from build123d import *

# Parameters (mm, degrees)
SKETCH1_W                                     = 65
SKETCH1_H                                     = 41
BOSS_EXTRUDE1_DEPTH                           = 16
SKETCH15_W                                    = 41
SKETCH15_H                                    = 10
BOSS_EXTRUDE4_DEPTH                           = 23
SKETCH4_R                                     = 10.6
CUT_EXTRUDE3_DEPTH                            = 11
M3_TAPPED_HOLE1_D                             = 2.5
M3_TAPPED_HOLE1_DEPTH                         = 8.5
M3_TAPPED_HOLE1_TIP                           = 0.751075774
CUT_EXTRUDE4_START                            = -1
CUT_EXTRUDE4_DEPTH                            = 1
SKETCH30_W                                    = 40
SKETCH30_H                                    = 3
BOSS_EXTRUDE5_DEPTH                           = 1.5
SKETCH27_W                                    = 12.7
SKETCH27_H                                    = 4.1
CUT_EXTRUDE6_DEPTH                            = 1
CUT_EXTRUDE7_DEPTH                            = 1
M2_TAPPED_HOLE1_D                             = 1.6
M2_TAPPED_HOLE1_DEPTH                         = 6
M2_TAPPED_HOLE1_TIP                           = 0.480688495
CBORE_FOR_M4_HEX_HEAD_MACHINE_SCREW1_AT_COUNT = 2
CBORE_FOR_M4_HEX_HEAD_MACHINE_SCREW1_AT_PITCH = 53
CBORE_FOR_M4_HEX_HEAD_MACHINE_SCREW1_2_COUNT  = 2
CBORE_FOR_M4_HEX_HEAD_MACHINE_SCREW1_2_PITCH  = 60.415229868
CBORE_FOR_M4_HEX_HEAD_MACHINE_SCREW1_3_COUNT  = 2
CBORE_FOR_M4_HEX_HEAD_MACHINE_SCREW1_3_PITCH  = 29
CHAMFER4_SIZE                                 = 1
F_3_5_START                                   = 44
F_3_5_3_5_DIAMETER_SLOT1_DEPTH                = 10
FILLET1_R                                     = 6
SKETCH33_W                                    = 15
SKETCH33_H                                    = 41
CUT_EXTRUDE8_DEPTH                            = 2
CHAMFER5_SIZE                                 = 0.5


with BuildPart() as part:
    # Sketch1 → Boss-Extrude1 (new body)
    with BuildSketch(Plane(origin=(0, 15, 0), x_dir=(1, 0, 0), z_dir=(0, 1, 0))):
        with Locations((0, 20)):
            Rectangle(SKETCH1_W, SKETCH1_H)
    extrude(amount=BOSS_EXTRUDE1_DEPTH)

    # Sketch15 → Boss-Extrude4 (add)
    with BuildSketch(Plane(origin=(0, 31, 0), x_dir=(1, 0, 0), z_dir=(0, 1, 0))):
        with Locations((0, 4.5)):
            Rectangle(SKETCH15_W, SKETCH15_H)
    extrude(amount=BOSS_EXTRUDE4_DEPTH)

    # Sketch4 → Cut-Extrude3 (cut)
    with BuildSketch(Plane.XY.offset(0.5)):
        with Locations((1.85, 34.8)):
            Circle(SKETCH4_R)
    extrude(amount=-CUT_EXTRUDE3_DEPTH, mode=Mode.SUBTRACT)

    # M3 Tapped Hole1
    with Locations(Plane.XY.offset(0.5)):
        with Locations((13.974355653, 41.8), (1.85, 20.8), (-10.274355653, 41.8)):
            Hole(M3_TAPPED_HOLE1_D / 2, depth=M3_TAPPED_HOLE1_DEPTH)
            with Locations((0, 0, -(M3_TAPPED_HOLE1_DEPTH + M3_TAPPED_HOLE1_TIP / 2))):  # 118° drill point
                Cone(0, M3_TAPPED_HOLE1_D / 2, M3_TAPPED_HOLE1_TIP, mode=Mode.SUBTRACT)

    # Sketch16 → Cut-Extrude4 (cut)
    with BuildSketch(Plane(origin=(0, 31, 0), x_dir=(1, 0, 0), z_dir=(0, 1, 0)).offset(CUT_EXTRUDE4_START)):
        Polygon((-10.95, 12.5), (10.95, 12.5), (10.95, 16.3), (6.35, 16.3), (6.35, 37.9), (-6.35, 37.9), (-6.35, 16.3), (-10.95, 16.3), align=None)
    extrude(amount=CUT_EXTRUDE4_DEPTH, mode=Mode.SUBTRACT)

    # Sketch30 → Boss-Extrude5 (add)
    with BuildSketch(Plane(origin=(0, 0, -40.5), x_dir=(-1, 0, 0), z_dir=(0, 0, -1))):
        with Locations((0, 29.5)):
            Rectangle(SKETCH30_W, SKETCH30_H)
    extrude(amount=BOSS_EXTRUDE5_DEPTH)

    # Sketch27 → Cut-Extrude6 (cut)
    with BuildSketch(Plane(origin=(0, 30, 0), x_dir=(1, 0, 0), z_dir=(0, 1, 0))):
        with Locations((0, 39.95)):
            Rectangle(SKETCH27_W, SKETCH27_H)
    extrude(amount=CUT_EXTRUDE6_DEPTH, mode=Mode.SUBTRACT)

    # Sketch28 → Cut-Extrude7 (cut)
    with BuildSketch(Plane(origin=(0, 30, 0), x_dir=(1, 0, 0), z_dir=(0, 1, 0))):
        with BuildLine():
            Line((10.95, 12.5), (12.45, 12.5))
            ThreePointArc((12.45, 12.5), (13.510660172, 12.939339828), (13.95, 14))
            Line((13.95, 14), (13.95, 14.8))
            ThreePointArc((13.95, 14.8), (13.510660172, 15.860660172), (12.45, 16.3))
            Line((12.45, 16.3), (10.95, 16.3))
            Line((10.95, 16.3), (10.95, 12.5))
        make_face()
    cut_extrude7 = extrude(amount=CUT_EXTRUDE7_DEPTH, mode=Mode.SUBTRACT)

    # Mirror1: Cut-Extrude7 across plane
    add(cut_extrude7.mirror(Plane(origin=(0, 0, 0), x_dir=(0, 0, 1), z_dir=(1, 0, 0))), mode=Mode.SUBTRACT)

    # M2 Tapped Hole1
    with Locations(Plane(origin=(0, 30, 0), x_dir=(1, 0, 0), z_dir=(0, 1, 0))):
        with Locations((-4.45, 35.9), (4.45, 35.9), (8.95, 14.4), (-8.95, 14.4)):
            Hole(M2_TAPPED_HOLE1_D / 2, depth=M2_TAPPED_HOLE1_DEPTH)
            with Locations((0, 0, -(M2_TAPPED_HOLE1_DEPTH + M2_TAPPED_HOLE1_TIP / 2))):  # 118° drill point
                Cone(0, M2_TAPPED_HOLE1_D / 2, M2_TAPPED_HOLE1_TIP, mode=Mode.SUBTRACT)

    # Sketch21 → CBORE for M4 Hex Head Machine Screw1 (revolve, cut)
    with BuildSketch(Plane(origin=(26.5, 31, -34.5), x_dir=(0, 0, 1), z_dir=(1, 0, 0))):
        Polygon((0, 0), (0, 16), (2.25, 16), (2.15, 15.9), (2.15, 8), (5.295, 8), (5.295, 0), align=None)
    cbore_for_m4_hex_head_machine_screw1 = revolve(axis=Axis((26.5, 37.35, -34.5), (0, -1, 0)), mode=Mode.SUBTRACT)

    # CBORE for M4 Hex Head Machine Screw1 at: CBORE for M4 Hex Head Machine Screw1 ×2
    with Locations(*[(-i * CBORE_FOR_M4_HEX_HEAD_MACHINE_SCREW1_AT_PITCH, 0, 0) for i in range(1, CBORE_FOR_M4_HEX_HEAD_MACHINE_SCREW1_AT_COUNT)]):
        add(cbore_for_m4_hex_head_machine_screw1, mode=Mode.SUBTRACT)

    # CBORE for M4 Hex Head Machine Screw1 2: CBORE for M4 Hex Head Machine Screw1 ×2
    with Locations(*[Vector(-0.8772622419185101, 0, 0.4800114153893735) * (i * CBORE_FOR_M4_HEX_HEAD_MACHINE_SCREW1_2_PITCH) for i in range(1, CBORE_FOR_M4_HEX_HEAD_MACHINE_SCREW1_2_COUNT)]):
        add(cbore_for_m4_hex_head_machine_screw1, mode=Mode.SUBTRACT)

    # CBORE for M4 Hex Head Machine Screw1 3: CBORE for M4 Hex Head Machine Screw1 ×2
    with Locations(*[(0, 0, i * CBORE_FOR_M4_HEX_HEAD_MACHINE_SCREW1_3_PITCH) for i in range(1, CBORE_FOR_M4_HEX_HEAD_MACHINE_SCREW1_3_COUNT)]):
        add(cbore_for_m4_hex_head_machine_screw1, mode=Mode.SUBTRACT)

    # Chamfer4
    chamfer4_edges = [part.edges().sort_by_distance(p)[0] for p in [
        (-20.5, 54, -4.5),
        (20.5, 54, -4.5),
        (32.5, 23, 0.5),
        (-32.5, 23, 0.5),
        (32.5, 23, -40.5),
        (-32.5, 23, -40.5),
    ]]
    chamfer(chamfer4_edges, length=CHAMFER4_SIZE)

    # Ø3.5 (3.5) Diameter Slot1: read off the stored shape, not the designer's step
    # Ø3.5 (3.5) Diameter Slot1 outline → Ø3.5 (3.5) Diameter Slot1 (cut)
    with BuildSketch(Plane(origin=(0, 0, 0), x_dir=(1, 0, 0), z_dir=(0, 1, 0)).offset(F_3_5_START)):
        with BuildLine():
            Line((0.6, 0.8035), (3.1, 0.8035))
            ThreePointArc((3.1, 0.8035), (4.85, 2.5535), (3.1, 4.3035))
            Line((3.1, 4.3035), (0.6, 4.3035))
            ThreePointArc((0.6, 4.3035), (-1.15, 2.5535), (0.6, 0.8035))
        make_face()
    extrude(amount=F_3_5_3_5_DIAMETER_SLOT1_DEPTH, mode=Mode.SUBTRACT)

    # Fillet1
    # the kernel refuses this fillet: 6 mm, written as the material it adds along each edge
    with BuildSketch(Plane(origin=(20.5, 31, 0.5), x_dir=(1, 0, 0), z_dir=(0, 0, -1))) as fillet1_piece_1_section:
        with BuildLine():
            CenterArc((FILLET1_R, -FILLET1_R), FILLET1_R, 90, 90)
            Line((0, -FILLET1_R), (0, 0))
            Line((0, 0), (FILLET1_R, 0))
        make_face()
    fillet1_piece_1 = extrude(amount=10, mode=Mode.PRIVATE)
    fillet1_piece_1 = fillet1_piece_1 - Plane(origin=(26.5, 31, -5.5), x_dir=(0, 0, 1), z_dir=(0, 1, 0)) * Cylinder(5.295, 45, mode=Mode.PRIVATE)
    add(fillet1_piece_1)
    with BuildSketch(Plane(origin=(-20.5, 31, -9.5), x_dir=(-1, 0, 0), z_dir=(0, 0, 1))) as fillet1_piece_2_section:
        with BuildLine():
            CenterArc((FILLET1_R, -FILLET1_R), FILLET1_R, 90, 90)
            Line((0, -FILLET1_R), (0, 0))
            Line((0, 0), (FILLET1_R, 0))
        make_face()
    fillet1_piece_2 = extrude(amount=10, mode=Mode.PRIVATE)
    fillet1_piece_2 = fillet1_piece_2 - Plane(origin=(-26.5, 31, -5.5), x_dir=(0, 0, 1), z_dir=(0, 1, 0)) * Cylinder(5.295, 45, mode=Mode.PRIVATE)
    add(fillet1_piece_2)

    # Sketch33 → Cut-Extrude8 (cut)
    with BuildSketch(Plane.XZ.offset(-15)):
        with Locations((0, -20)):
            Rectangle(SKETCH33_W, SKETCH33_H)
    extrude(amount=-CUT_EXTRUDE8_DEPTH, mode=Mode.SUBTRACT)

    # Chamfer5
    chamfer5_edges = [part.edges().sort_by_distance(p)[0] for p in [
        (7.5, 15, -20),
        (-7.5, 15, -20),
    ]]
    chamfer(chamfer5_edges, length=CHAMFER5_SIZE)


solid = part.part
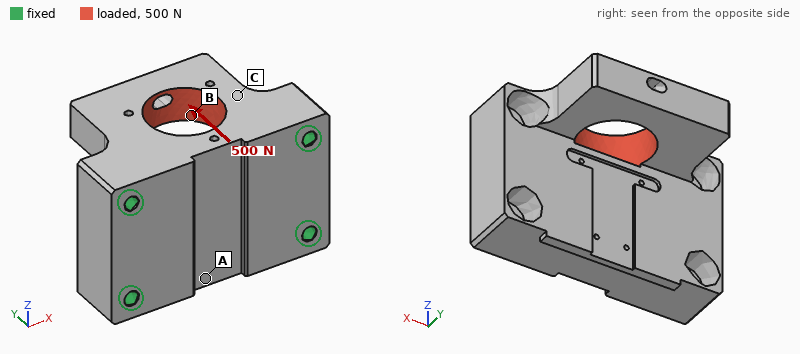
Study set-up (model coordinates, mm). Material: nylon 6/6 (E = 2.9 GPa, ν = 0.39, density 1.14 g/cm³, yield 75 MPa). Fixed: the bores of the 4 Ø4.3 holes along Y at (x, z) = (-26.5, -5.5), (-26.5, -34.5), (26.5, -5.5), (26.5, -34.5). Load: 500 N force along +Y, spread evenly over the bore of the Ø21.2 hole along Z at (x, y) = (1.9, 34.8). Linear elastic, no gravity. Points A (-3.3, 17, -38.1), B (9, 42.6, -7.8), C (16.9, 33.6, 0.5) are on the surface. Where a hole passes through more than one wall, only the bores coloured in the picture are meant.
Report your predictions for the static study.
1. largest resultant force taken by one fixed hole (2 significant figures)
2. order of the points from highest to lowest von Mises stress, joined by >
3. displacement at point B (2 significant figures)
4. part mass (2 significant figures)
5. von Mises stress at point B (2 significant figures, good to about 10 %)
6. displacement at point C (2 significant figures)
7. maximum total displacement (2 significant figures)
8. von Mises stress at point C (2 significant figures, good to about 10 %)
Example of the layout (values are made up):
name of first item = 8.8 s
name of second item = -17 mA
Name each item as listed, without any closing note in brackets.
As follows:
largest resultant force taken by one fixed hole = 290 N
order of the points from highest to lowest von Mises stress, joined by > = B > C > A
displacement at point B = 37 µm
part mass = 49 g
von Mises stress at point B = 2.9 MPa
displacement at point C = 38 µm
maximum total displacement = 53 µm
von Mises stress at point C = 2.0 MPa
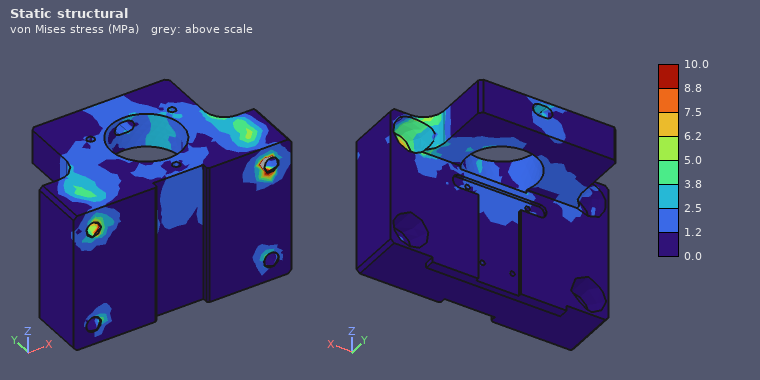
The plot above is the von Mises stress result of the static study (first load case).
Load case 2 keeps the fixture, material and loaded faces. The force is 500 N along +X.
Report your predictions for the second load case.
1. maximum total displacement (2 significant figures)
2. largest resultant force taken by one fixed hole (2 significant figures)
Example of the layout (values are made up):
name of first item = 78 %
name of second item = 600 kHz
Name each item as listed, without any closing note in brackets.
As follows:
maximum total displacement = 61 µm
largest resultant force taken by one fixed hole = 220 N
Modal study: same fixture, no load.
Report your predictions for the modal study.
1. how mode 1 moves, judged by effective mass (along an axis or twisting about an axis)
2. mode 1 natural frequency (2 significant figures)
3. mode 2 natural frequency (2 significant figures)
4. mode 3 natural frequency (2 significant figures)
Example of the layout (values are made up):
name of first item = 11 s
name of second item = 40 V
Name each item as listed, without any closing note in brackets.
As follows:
how mode 1 moves, judged by effective mass = along Z
mode 1 natural frequency = 2300 Hz
mode 2 natural frequency = 4000 Hz
mode 3 natural frequency = 4100 Hz
